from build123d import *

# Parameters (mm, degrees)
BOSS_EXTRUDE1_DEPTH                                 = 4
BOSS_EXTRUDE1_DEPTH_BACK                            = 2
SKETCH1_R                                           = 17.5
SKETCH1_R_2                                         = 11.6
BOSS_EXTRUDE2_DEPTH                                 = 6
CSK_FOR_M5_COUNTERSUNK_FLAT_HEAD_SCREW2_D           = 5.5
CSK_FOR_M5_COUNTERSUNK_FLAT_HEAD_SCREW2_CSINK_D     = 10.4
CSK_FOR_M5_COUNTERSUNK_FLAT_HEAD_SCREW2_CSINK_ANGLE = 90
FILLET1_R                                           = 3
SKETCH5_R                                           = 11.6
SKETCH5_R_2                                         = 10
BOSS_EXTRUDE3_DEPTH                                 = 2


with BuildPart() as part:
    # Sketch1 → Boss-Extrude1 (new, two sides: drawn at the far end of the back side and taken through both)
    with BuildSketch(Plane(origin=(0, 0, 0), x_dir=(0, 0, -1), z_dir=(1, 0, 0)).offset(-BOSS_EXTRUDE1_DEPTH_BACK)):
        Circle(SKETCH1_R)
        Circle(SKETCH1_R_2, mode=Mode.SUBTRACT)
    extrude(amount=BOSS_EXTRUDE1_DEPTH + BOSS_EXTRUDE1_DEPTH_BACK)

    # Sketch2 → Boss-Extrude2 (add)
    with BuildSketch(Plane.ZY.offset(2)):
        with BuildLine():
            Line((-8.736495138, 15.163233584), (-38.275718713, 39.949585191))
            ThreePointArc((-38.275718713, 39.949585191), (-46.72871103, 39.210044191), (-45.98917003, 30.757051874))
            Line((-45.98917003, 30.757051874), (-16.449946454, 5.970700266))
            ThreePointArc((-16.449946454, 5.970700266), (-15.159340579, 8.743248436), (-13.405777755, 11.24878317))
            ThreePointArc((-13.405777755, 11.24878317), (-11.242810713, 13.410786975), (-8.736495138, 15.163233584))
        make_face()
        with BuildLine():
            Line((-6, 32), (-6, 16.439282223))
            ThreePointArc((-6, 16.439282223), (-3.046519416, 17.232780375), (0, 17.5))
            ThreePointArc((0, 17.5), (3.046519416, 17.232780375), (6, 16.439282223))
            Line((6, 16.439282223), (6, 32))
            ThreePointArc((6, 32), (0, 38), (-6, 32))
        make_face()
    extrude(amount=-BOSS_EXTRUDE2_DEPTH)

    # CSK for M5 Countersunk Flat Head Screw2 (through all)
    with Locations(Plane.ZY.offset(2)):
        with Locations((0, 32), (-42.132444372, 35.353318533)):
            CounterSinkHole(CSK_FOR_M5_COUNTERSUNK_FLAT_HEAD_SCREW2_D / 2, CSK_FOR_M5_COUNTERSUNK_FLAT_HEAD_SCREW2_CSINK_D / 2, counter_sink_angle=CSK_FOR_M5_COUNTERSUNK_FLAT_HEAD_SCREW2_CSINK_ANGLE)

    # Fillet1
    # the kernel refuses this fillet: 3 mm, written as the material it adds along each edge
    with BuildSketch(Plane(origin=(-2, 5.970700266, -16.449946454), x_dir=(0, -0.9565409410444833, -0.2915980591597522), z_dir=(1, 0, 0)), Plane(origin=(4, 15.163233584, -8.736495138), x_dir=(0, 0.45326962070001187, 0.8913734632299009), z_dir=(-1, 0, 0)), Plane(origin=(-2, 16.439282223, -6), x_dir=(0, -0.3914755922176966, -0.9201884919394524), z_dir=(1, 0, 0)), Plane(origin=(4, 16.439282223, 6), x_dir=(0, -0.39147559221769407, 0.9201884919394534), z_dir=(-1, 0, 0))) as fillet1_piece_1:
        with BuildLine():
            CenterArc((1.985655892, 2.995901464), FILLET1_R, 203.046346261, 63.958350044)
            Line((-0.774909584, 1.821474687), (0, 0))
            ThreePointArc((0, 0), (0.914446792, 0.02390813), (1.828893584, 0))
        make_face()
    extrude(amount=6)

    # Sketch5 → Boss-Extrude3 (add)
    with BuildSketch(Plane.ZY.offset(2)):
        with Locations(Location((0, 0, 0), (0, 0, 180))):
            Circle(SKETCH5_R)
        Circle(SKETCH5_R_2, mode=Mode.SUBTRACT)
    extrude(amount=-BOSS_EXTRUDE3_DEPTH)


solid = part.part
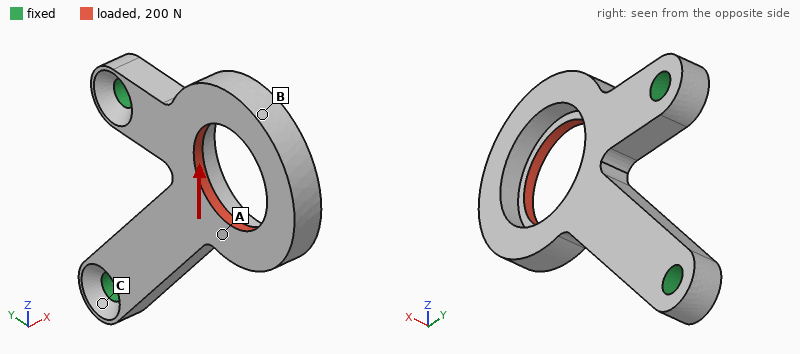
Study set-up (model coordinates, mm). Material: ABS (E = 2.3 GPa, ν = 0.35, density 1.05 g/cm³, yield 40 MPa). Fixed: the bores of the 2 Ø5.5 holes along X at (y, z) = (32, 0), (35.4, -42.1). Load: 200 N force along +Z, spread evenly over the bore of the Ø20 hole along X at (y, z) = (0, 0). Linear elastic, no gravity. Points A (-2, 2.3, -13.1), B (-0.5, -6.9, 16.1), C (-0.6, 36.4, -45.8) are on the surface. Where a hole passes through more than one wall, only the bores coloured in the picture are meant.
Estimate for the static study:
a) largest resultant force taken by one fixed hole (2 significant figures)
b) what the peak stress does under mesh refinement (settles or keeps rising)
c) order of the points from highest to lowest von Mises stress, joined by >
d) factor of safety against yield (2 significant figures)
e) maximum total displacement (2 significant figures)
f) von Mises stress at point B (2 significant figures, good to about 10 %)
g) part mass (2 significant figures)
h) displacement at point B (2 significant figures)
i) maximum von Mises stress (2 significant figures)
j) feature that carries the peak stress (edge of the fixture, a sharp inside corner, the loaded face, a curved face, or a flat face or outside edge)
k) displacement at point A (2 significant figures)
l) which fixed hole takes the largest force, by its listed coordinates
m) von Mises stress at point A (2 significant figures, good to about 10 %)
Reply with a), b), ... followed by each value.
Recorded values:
a) 220 N
b) settles
c) A > B > C
d) 1.7
e) 0.47 mm
f) 5.5 MPa
g) 7.9 g
h) 0.45 mm
i) 23 MPa
j) a curved face
k) 0.16 mm
l) (35.4, -42.1)
m) 9.3 MPa
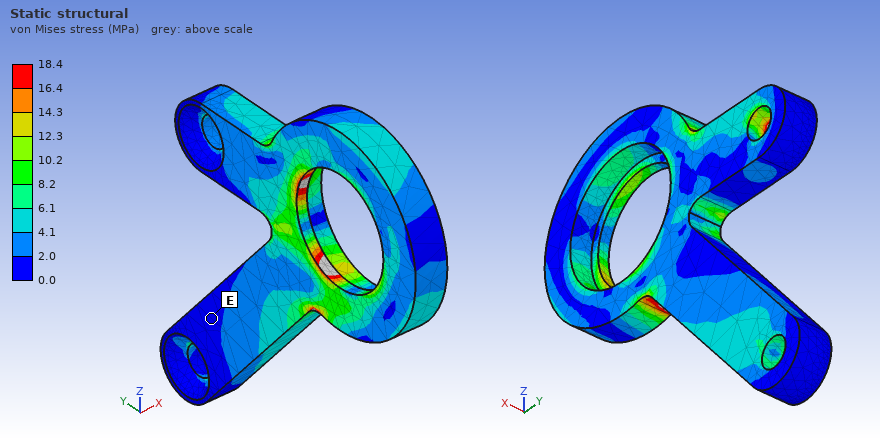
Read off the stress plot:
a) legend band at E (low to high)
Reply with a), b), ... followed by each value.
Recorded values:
a) 0.0 to 2.0 MPa
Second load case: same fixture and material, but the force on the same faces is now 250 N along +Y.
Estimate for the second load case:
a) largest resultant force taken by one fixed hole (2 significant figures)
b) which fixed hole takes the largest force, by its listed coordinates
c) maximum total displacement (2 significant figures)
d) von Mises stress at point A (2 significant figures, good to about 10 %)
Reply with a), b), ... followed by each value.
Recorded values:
a) 240 N
b) (32, 0)
c) 0.92 mm
d) 5.5 MPa
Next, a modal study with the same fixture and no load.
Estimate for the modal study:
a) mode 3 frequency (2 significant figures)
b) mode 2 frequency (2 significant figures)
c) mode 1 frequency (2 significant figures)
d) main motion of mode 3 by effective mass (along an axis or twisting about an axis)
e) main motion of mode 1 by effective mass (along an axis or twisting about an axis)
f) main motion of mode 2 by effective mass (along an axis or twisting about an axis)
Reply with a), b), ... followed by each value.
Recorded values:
a) 1900 Hz
b) 1400 Hz
c) 530 Hz
d) along Z
e) along X
f) twisting about Y
